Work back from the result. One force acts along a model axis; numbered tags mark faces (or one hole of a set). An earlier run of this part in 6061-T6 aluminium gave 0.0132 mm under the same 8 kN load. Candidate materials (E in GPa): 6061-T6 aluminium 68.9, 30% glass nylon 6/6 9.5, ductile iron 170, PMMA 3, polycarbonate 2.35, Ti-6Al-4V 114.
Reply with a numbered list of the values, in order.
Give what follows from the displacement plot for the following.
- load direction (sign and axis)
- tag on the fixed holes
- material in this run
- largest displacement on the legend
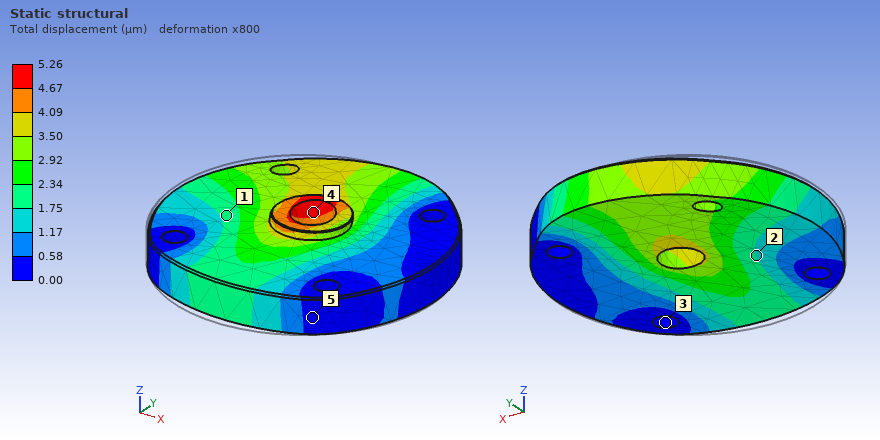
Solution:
1. +Y
2. 3
3. ductile iron
4. 5.26 µm
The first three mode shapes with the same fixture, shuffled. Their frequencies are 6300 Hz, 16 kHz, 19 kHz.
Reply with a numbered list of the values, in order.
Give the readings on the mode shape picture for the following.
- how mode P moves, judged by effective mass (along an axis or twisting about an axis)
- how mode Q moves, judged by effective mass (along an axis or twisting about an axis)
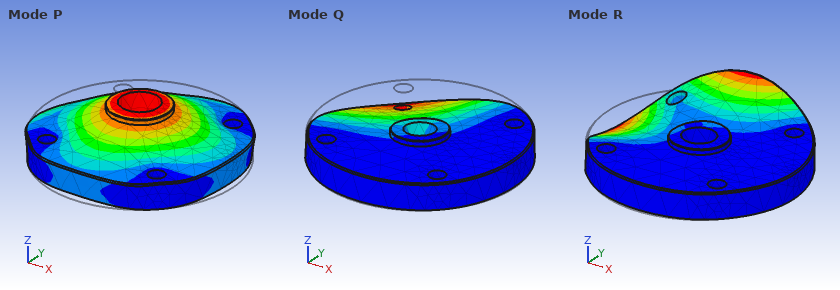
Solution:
1. along Z
2. along Z
